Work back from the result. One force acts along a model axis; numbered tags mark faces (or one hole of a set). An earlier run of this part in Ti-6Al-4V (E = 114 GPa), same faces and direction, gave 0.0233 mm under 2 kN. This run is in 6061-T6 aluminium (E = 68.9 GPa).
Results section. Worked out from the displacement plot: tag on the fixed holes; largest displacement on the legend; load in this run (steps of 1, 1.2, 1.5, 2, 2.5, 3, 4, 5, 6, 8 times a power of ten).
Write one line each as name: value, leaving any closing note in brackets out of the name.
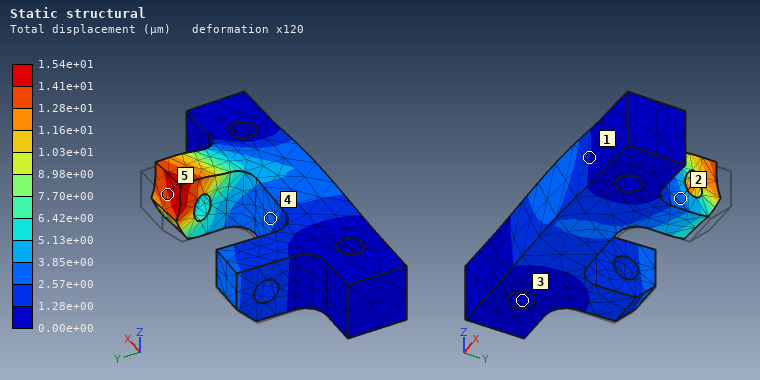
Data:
tag on the fixed holes: 3
largest displacement on the legend: 1.54e+01 µm
load in this run: 800 N
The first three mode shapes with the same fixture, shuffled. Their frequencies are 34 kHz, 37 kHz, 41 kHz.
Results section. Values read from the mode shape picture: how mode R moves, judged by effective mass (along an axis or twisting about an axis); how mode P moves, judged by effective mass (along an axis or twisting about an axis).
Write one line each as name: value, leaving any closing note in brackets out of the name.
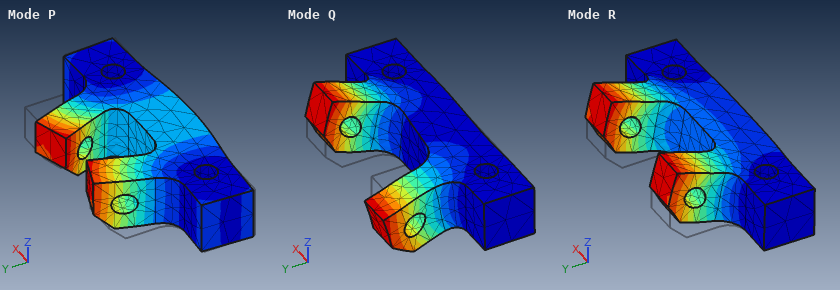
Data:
how mode R moves, judged by effective mass: along Z
how mode P moves, judged by effective mass: along Y
